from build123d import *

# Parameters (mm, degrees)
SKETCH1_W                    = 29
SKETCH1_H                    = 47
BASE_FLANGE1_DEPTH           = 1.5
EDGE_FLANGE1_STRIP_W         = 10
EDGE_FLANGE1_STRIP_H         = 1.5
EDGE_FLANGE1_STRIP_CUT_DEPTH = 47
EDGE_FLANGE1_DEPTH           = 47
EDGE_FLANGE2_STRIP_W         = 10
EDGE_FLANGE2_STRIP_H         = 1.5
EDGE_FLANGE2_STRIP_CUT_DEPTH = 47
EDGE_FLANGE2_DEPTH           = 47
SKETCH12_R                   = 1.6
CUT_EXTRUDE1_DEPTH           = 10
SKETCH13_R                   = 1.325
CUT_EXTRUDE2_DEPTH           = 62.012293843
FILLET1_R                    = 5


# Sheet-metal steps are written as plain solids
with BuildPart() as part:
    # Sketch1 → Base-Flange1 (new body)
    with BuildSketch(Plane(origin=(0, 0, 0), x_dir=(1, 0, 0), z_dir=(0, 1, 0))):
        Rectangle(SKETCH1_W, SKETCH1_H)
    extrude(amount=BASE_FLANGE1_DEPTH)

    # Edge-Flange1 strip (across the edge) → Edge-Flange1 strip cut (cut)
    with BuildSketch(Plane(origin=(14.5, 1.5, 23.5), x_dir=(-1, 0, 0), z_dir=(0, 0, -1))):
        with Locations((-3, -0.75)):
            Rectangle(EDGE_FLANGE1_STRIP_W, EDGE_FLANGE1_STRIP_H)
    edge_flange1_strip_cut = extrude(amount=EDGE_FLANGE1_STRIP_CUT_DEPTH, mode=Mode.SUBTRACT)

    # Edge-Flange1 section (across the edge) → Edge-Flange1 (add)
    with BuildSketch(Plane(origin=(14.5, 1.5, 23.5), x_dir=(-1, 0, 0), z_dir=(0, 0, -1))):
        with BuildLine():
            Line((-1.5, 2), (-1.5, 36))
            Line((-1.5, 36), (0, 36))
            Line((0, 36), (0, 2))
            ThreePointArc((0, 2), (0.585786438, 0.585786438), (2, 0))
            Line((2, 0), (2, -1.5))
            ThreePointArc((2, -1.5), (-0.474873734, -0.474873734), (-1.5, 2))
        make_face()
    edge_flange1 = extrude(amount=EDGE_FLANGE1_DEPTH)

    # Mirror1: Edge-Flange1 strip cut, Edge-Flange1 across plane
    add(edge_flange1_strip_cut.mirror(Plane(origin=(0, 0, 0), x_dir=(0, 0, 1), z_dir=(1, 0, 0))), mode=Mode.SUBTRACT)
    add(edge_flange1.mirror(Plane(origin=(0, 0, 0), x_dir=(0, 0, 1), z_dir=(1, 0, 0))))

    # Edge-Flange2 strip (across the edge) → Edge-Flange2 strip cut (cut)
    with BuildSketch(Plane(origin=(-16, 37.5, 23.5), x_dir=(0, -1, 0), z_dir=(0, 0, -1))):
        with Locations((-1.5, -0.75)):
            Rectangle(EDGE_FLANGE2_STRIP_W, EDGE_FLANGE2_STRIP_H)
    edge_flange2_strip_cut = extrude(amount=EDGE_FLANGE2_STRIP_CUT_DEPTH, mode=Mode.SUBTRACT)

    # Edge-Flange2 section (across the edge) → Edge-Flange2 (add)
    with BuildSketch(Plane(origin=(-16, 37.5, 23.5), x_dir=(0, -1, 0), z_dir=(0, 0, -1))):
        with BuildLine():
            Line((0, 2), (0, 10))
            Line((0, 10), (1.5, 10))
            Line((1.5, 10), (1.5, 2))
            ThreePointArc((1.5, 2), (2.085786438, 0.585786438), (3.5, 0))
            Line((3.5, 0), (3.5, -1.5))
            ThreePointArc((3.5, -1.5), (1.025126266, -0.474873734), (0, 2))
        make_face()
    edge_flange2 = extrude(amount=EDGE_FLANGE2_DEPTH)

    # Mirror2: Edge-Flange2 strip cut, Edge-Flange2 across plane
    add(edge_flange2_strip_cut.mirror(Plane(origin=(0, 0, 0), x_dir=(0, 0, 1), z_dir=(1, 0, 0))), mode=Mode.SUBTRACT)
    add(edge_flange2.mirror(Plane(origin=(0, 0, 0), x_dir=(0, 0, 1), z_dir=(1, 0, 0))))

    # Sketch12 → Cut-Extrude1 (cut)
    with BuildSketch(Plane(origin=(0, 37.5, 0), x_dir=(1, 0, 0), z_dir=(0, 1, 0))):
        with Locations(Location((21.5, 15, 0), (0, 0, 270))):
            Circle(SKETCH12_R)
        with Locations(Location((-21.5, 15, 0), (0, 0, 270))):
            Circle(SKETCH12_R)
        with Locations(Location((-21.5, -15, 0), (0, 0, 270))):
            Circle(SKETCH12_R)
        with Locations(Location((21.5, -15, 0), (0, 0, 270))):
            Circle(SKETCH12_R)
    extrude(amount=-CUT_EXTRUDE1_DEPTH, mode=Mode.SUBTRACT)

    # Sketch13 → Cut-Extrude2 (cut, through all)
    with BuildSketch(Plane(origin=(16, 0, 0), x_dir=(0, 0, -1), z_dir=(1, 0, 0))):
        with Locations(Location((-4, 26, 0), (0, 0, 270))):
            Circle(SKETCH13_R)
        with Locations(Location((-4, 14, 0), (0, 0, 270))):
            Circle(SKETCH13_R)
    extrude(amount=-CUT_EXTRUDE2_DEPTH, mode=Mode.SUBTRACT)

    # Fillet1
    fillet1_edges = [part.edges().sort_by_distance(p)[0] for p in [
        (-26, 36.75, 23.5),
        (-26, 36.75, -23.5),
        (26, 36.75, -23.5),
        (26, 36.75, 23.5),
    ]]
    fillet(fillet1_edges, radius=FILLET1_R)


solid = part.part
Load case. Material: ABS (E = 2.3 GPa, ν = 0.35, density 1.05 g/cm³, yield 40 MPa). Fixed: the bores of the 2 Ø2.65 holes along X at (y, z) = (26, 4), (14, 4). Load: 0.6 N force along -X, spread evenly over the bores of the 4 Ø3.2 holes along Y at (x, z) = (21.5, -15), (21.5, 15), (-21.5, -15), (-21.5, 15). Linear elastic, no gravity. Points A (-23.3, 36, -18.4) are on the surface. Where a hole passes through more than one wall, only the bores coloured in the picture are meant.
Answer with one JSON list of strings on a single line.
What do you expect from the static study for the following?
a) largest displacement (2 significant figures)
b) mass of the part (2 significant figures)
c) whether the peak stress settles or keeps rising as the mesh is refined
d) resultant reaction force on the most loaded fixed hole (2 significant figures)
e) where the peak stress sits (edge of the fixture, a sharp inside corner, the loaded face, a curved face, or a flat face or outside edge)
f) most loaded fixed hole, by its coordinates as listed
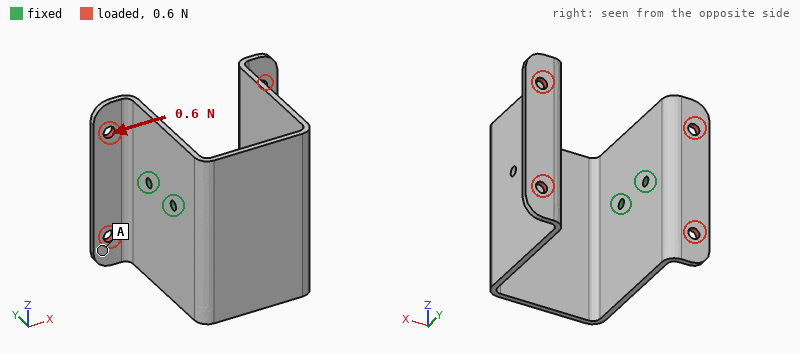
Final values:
["0.76 mm", "8.7 g", "keeps rising", "0.73 N", "edge of the fixture", "(26, 4)"]
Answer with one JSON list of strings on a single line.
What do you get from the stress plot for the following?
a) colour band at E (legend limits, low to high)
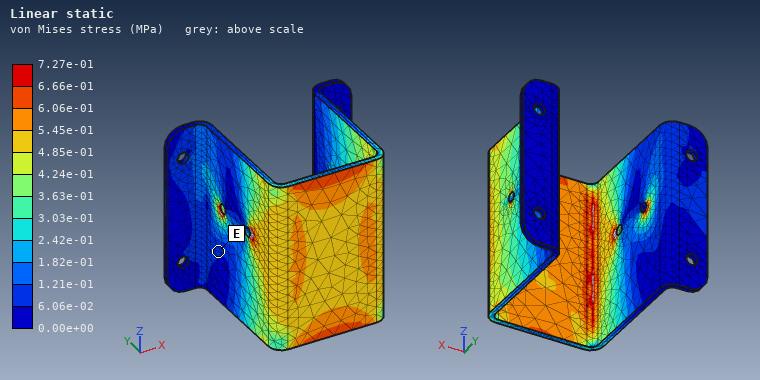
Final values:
["6.06e-02 to 1.21e-01 MPa"]
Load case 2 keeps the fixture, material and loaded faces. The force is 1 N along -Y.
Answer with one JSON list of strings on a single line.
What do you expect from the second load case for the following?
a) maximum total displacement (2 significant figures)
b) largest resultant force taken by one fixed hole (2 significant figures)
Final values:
["0.93 mm", "0.88 N"]
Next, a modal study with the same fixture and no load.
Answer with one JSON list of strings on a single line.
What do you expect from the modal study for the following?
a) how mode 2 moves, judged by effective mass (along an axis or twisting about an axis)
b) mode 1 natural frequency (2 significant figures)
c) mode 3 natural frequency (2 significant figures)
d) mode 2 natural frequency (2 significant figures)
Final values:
["along Z", "70 Hz", "190 Hz", "96 Hz"]
